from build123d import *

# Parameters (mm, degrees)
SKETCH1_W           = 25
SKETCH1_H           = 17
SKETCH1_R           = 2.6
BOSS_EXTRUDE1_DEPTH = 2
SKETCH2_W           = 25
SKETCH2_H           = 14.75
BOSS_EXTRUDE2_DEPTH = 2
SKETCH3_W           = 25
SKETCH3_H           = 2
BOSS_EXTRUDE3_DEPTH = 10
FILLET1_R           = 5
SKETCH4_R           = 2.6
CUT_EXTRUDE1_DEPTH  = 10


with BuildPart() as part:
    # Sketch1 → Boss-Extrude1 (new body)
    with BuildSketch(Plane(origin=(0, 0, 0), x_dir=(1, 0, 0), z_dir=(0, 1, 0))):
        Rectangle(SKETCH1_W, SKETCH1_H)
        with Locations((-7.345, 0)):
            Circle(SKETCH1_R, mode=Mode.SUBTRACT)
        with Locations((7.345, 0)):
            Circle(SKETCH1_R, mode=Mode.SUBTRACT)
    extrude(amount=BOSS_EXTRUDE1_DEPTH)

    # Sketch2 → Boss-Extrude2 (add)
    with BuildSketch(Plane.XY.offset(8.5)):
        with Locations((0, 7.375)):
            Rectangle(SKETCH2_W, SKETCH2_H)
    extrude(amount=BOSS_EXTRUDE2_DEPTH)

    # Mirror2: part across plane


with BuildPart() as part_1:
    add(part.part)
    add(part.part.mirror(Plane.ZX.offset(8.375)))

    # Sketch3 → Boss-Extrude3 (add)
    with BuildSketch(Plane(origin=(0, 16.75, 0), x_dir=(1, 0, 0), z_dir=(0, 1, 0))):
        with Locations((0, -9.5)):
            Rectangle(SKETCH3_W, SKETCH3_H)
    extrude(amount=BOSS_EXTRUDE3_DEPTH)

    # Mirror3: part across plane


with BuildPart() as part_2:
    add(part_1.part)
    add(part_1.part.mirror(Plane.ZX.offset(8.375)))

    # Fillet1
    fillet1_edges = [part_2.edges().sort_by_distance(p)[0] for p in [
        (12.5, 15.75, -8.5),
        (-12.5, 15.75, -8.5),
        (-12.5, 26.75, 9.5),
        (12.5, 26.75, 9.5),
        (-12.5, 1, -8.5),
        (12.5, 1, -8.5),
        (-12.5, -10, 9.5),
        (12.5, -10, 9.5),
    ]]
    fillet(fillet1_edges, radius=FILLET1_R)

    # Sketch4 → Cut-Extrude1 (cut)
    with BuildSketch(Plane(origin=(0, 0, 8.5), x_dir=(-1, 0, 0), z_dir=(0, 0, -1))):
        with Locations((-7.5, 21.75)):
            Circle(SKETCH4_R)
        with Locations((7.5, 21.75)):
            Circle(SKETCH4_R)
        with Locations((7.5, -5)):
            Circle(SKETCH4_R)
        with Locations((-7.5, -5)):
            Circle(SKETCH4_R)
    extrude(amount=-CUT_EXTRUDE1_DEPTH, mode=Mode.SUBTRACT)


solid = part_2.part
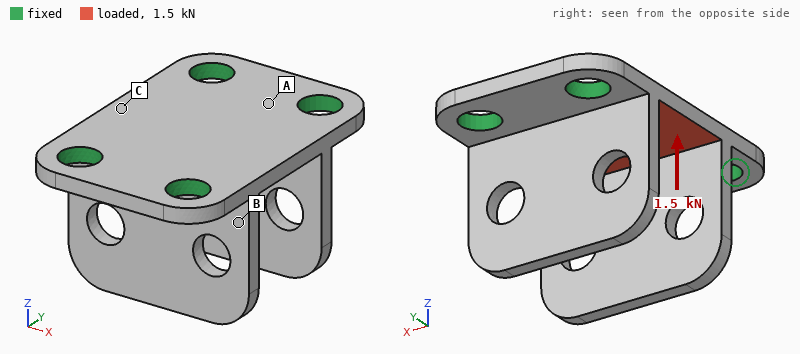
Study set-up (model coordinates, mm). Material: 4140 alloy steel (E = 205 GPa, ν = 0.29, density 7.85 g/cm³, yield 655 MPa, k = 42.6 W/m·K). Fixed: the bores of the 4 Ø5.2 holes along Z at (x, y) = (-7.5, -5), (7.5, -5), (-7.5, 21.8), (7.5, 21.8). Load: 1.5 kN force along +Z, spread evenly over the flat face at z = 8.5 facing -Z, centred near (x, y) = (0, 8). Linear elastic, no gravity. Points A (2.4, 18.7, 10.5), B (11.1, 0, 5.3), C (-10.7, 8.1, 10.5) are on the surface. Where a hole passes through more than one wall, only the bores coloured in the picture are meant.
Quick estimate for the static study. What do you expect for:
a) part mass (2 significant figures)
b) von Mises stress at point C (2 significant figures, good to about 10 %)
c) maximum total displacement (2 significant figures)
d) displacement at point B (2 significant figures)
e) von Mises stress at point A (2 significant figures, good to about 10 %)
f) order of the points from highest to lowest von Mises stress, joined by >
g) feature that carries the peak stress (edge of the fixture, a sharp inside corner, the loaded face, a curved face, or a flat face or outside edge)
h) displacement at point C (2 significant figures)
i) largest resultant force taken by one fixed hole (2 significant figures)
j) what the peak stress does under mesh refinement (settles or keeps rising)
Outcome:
24 g
140 MPa
52 µm
13 µm
91 MPa
C > A > B
edge of the fixture
24 µm
380 N
keeps rising
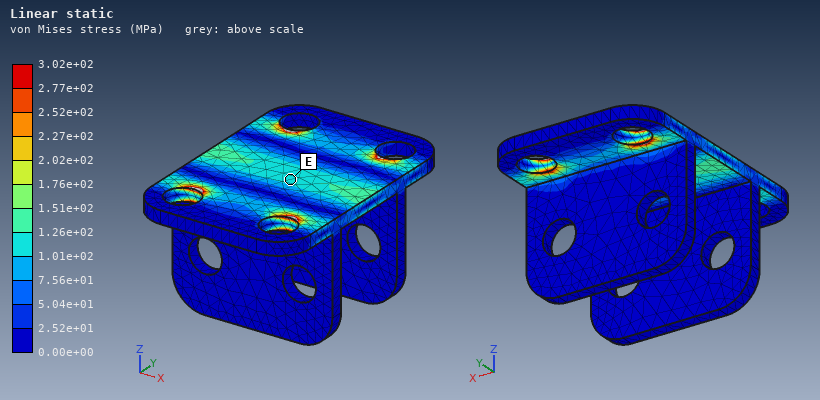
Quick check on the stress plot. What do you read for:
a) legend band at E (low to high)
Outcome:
1.01e+02 to 1.26e+02 MPa
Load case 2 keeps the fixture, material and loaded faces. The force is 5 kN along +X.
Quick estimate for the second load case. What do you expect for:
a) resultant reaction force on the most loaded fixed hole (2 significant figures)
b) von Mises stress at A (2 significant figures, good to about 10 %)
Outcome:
1.4 kN
76 MPa
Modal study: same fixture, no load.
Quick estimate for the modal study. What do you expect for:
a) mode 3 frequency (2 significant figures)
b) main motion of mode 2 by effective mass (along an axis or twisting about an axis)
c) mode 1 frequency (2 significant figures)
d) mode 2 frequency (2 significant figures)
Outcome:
9300 Hz
along Y
4400 Hz
5100 Hz
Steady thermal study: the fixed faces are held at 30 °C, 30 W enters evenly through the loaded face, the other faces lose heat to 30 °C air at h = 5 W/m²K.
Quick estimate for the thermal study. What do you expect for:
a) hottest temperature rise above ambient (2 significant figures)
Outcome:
62 K
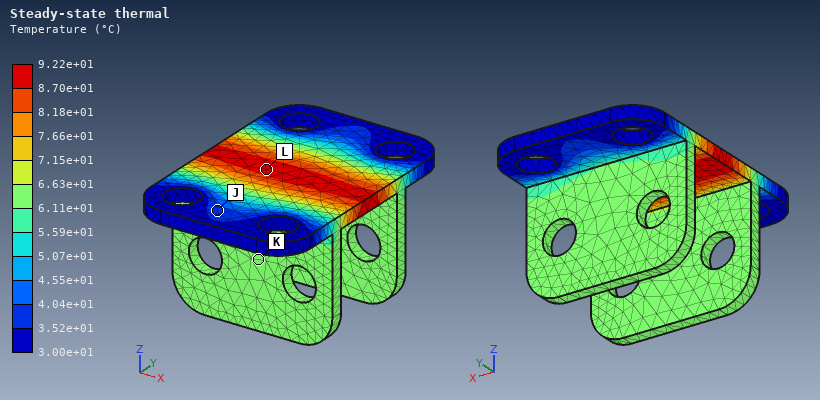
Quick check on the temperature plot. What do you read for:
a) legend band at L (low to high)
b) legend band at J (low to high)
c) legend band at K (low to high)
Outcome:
8.70e+01 to 9.22e+01 °C
3.52e+01 to 4.04e+01 °C
6.11e+01 to 6.63e+01 °C
